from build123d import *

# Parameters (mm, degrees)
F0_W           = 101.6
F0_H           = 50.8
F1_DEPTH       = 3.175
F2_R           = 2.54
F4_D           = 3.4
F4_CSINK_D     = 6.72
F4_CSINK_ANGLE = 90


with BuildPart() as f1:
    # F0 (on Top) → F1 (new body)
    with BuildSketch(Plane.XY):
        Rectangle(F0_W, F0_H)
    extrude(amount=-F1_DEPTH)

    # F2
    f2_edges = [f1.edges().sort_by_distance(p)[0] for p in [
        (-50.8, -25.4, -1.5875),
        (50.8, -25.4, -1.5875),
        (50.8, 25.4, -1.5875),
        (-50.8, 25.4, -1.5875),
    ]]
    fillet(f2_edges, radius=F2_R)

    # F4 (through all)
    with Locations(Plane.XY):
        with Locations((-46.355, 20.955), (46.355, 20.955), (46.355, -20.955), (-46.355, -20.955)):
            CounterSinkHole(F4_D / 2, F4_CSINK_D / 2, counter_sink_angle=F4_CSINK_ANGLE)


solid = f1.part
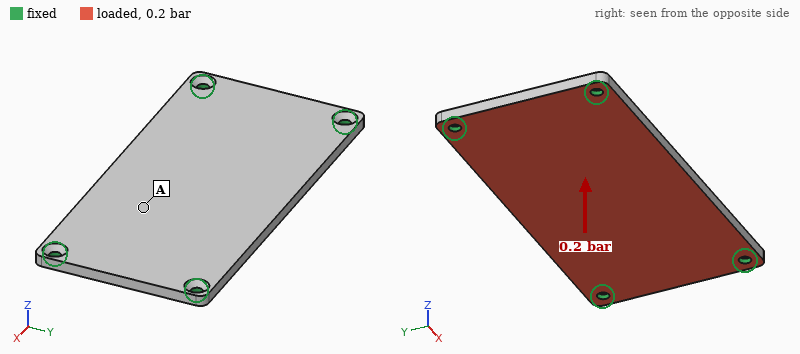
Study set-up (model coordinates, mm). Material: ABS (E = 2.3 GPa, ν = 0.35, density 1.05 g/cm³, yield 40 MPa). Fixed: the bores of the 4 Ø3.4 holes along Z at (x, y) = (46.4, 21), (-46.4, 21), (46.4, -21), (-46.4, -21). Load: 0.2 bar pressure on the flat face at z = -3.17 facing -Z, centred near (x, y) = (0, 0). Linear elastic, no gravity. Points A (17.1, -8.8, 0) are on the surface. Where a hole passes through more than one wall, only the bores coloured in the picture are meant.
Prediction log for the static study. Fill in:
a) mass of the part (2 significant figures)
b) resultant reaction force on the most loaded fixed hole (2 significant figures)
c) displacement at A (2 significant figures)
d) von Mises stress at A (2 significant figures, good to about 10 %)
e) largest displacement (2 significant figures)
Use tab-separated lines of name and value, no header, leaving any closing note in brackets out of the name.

mass of the part	17 g
resultant reaction force on the most loaded fixed hole	46 N
displacement at A	0.81 mm
von Mises stress at A	4.0 MPa
largest displacement	1.1 mm
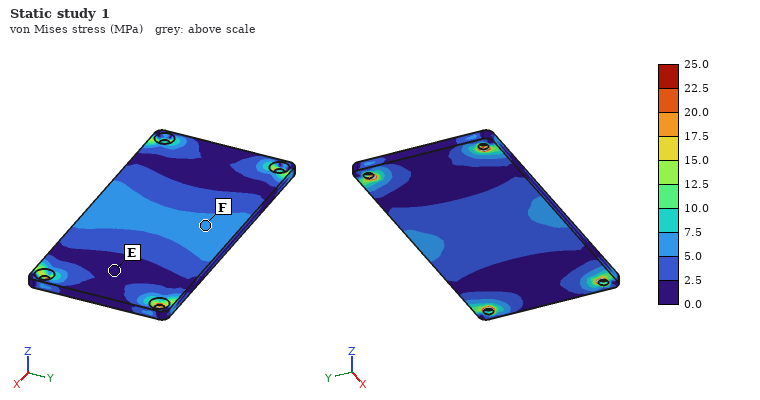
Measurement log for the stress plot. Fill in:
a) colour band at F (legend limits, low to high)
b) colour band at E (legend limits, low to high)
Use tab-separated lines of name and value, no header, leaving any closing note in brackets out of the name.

colour band at F	5.0 to 7.5 MPa
colour band at E	0.0 to 2.5 MPa
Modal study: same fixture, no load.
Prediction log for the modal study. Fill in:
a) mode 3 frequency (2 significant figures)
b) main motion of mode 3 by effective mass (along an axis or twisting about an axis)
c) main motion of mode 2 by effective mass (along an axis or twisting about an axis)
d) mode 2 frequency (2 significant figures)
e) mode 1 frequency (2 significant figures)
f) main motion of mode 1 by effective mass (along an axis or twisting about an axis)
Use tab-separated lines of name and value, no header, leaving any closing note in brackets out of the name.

mode 3 frequency	1200 Hz
main motion of mode 3 by effective mass	twisting about Y
main motion of mode 2 by effective mass	twisting about X
mode 2 frequency	810 Hz
mode 1 frequency	440 Hz
main motion of mode 1 by effective mass	along Z
